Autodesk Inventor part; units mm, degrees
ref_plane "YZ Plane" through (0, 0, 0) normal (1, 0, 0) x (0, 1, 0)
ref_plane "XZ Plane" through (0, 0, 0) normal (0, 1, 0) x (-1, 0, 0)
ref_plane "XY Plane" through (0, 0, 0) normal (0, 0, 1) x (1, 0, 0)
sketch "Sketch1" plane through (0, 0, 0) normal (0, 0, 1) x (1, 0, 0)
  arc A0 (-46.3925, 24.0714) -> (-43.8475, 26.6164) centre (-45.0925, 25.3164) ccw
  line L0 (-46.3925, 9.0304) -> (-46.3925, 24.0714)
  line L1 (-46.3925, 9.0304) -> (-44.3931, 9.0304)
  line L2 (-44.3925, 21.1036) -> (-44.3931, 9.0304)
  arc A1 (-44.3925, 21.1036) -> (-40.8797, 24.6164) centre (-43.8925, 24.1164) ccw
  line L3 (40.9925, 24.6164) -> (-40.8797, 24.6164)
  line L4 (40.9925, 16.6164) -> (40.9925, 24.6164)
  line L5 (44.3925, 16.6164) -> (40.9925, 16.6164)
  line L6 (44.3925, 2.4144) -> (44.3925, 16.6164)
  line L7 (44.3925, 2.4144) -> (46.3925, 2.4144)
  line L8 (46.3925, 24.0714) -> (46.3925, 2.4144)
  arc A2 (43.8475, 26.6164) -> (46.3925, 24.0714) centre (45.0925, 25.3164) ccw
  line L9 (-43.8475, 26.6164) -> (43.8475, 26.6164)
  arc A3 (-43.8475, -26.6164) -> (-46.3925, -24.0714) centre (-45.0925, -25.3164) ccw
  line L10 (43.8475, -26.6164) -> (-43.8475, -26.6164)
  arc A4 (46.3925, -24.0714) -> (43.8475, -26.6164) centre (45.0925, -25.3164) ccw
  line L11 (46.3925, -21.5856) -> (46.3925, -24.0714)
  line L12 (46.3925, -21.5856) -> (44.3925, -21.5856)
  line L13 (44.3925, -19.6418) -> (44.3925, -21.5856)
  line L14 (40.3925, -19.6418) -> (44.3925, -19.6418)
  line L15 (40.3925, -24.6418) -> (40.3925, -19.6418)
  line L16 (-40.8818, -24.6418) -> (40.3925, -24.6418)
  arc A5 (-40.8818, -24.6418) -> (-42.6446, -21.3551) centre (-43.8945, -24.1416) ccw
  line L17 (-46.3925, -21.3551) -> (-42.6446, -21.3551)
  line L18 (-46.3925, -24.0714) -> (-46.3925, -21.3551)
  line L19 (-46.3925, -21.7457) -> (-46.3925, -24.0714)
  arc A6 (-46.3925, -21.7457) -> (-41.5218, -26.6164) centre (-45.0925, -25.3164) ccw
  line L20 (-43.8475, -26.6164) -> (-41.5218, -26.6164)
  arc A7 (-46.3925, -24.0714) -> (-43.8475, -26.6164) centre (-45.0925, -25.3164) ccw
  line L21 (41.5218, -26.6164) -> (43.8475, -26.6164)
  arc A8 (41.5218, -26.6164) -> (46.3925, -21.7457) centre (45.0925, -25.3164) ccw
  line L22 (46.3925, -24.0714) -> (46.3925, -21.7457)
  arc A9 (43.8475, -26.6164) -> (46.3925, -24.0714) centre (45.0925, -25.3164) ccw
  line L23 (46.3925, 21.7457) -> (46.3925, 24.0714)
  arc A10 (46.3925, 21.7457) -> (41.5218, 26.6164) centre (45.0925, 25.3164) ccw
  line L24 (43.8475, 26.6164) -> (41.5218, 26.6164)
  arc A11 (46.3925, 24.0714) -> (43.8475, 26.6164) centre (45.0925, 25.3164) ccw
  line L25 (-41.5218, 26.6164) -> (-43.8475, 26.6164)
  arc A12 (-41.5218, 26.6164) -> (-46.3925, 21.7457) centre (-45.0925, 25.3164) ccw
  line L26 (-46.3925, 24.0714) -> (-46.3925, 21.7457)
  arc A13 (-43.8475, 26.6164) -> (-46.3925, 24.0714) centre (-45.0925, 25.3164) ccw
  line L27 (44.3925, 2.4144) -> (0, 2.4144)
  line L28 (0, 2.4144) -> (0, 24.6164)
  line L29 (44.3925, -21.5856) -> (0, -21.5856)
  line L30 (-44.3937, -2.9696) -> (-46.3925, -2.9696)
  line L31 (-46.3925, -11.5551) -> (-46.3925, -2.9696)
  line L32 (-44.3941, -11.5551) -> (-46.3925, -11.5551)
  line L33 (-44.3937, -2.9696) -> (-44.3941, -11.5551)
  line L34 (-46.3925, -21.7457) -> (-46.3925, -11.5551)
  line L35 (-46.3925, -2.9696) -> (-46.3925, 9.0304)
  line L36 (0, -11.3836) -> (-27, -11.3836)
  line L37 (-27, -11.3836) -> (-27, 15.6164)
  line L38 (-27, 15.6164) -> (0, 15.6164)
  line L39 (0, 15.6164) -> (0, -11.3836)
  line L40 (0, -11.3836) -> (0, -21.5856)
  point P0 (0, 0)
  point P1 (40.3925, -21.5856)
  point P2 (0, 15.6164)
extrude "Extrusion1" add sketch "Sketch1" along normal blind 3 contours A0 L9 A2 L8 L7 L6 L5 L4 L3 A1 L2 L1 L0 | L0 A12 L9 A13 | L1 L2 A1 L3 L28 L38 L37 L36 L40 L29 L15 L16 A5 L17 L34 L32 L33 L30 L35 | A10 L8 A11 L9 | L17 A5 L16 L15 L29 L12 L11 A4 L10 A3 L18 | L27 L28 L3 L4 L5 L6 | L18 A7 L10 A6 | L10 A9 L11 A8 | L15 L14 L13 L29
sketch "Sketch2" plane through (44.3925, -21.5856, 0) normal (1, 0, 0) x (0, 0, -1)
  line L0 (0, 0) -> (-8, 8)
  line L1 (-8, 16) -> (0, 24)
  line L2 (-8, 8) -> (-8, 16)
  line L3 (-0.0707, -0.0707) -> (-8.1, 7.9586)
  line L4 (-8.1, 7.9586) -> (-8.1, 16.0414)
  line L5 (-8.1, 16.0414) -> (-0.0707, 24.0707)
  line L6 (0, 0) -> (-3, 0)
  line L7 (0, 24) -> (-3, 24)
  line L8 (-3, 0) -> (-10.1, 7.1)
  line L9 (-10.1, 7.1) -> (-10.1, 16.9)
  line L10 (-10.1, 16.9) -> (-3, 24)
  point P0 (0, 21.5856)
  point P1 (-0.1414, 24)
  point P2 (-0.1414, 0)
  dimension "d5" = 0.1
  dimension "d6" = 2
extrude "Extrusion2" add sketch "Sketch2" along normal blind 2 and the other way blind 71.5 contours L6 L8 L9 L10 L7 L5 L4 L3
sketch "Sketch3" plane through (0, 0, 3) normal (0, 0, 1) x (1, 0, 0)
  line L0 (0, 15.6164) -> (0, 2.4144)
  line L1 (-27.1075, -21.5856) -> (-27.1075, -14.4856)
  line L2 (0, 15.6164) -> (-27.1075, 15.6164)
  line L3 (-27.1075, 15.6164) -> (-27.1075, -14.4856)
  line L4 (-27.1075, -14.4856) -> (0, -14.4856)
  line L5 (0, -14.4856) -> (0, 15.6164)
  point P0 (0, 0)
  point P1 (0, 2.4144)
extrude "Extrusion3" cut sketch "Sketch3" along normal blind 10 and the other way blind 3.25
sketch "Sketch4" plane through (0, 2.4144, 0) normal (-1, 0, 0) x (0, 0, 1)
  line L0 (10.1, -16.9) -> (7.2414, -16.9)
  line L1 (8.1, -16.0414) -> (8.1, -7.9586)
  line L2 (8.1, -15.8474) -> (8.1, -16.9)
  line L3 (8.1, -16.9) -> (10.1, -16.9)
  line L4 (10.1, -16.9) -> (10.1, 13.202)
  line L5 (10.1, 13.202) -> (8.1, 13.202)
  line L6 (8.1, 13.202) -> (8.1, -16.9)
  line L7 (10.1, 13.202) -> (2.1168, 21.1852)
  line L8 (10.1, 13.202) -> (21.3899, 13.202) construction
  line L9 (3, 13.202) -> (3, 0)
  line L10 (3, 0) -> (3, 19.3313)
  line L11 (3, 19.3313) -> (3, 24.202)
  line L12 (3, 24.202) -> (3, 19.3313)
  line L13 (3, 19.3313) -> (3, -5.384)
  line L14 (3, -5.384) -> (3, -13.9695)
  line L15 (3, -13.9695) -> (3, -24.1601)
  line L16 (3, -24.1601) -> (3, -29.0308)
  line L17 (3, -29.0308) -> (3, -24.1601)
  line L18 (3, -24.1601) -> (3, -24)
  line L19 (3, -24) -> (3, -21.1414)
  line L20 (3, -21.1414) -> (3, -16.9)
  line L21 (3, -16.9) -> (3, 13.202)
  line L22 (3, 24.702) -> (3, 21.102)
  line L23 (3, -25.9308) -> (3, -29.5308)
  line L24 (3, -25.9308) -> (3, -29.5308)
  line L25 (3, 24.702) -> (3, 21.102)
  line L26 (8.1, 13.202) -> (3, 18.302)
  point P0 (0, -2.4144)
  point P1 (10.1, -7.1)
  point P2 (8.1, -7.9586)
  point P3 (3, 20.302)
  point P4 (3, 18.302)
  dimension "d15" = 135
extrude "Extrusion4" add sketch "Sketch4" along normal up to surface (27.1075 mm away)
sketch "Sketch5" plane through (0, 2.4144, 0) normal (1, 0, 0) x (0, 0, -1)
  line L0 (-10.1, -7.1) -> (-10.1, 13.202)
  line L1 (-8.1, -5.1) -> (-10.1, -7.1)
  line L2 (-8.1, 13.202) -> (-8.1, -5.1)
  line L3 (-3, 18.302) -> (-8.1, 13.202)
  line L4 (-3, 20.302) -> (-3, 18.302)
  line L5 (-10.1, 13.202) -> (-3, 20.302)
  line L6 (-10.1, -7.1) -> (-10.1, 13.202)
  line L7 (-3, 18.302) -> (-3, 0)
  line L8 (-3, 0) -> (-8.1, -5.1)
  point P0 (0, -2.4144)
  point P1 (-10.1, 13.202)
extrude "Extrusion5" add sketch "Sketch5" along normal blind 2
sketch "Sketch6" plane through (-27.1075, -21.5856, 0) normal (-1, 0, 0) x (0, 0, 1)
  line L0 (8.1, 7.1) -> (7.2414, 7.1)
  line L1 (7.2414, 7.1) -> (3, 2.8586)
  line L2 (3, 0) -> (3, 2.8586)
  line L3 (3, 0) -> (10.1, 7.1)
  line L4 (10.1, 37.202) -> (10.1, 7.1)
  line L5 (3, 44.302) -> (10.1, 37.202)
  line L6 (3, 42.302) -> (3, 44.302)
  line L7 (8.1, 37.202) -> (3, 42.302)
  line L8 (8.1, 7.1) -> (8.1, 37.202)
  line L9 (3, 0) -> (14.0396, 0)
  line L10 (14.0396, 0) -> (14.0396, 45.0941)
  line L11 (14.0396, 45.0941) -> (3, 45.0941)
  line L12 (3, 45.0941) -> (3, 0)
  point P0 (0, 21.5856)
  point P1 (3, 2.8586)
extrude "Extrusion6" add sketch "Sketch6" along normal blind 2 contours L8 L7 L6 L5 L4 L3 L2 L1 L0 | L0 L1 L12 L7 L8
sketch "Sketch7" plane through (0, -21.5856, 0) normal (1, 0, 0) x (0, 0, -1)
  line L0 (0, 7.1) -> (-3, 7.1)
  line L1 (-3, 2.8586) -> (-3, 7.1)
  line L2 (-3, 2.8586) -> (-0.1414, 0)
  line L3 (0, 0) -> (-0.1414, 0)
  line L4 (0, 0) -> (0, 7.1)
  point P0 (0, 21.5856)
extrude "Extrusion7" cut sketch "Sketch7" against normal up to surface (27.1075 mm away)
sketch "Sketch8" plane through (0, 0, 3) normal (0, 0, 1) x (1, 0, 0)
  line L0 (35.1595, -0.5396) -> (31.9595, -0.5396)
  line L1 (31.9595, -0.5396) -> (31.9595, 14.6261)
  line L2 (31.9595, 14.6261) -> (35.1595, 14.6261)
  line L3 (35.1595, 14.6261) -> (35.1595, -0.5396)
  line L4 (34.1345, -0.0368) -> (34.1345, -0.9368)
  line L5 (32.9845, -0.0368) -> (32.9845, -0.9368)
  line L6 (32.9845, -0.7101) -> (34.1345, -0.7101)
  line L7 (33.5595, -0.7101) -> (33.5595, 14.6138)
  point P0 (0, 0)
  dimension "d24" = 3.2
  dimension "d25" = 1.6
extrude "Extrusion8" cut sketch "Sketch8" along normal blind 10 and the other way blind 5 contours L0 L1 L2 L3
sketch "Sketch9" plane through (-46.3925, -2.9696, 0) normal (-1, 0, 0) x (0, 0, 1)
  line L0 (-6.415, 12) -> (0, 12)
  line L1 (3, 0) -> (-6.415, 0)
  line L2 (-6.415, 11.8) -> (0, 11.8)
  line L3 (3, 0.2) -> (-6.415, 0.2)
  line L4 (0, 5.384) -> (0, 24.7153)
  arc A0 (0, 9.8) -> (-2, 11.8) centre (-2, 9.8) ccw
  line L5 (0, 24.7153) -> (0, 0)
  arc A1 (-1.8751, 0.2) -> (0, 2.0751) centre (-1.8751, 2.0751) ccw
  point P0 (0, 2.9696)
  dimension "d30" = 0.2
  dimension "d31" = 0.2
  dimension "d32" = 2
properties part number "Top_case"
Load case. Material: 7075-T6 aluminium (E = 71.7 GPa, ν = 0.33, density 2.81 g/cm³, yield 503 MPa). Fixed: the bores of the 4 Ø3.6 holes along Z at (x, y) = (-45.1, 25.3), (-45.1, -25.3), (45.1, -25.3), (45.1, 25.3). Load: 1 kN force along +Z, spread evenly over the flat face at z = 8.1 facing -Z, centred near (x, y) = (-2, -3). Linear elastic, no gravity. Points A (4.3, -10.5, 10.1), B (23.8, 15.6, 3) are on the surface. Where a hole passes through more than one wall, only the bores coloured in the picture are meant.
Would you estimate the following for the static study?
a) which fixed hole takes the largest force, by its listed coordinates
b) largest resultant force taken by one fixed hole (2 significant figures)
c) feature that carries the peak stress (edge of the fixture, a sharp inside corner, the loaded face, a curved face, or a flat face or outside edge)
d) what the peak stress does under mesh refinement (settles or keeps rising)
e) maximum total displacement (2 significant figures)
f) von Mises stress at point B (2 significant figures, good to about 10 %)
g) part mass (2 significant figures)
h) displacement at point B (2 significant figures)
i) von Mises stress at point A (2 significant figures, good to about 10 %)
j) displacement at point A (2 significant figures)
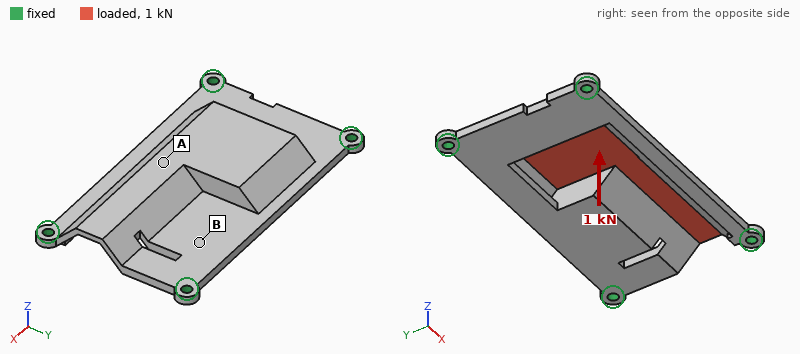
(45.1, -25.3)
840 N
edge of the fixture
keeps rising
0.17 mm
22 MPa
41 g
0.099 mm
41 MPa
0.12 mm
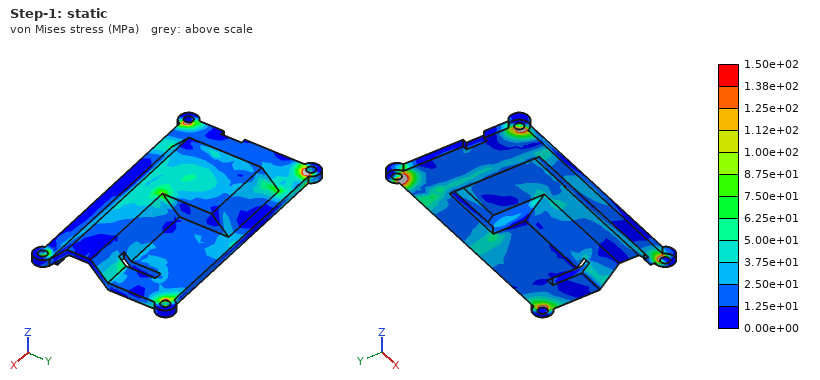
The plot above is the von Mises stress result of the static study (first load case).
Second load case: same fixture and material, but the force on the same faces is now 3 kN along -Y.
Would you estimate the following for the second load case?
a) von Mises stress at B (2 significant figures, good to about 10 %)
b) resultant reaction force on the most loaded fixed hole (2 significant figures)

40 MPa
1.2 kN
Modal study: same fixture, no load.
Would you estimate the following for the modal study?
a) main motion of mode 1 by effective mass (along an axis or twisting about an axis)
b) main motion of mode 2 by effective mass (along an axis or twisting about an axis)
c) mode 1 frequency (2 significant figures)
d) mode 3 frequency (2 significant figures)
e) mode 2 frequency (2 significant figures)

along Z
along Z
2400 Hz
4700 Hz
3600 Hz
